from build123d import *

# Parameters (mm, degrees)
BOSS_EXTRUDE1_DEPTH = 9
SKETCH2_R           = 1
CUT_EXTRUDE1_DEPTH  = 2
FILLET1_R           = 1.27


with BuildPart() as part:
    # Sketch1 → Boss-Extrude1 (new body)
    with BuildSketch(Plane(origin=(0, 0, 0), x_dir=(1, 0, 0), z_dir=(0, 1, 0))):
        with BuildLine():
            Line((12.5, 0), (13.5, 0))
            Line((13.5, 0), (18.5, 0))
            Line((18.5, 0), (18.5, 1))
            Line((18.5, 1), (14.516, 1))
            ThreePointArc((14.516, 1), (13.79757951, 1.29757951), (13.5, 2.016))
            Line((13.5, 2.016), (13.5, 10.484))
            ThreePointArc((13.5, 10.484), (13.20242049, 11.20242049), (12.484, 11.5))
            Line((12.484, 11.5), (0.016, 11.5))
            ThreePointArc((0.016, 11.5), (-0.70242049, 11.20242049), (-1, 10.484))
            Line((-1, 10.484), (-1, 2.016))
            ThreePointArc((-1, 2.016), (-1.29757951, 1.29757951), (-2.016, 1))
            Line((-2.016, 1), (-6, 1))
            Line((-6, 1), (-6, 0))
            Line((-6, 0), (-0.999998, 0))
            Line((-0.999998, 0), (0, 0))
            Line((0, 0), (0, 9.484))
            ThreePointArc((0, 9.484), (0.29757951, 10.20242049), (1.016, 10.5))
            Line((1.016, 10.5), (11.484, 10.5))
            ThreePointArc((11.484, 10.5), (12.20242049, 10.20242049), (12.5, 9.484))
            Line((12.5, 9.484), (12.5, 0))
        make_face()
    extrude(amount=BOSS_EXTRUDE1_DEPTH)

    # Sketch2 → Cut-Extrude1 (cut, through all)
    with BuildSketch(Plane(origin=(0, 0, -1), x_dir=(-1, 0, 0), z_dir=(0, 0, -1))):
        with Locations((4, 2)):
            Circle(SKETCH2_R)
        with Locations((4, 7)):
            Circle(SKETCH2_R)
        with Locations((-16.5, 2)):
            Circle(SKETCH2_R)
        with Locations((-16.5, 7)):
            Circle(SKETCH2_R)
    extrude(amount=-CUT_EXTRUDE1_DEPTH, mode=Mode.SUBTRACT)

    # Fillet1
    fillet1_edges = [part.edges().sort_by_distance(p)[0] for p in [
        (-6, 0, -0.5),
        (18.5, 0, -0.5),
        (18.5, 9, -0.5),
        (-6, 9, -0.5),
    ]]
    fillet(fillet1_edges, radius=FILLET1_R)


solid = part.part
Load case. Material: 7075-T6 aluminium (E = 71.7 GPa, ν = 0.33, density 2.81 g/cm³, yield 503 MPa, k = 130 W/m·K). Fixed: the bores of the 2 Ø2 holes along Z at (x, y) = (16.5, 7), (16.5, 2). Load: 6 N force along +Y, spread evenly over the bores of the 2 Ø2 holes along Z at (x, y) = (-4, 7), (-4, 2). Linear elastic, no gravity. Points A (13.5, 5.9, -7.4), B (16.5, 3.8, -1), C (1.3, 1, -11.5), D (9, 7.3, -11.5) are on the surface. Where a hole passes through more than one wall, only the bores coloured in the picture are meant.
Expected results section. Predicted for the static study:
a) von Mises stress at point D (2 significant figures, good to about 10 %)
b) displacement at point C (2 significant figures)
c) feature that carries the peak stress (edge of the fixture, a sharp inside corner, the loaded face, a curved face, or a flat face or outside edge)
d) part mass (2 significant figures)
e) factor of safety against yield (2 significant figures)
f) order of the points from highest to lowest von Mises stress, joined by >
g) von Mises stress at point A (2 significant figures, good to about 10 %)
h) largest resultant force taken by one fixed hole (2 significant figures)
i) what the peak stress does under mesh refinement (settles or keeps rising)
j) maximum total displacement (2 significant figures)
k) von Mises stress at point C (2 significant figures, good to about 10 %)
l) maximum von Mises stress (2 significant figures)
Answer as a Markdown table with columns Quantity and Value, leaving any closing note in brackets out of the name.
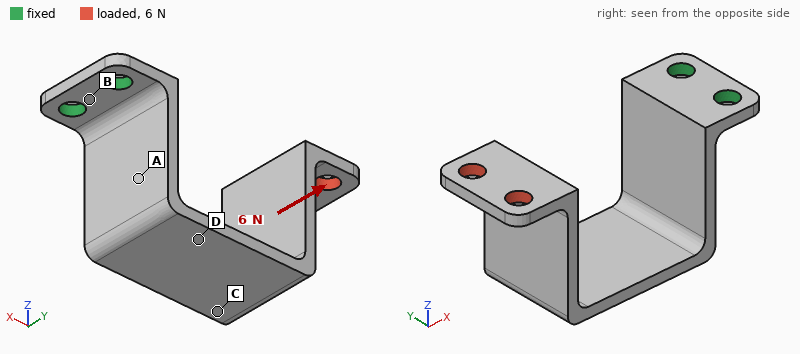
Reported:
| Quantity | Value |
|---|---|
| von Mises stress at point D | 38 MPa |
| displacement at point C | 0.12 mm |
| feature that carries the peak stress | a curved face |
| part mass | 1.1 g |
| factor of safety against yield | 7.9 |
| order of the points from highest to lowest von Mises stress, joined by > | A > D > C > B |
| von Mises stress at point A | 53 MPa |
| largest resultant force taken by one fixed hole | 20 N |
| what the peak stress does under mesh refinement | settles |
| maximum total displacement | 0.32 mm |
| von Mises stress at point C | 27 MPa |
| maximum von Mises stress | 63 MPa |
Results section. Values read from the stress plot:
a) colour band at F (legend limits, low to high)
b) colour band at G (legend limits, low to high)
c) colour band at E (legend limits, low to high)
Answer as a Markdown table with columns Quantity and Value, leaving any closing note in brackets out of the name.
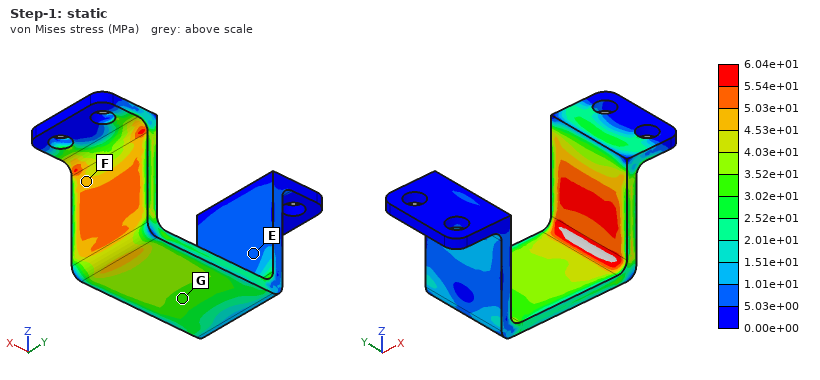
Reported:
| Quantity | Value |
|---|---|
| colour band at F | 4.53e+01 to 5.03e+01 MPa |
| colour band at G | 3.02e+01 to 3.52e+01 MPa |
| colour band at E | 5.03e+00 to 1.01e+01 MPa |
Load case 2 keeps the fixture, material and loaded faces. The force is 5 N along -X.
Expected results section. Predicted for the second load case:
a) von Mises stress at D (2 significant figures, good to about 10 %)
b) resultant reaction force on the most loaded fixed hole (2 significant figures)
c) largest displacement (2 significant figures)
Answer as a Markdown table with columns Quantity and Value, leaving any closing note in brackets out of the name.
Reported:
| Quantity | Value |
|---|---|
| von Mises stress at D | 33 MPa |
| resultant reaction force on the most loaded fixed hole | 2.5 N |
| largest displacement | 0.31 mm |
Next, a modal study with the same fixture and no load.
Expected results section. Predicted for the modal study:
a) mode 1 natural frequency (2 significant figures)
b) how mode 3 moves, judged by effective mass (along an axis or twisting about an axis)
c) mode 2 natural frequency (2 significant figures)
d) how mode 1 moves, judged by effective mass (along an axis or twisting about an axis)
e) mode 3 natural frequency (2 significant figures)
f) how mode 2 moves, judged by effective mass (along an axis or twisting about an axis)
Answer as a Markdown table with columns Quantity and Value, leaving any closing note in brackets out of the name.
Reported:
| Quantity | Value |
|---|---|
| mode 1 natural frequency | 870 Hz |
| how mode 3 moves, judged by effective mass | along X |
| mode 2 natural frequency | 1400 Hz |
| how mode 1 moves, judged by effective mass | along Z |
| mode 3 natural frequency | 2000 Hz |
| how mode 2 moves, judged by effective mass | along Y |
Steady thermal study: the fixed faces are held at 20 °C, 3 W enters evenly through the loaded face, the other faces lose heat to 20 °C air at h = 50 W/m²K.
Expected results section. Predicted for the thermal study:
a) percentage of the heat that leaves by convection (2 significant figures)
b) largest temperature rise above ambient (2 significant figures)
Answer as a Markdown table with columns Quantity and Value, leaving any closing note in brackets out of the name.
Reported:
| Quantity | Value |
|---|---|
| percentage of the heat that leaves by convection | 43 % |
| largest temperature rise above ambient | 69 K |
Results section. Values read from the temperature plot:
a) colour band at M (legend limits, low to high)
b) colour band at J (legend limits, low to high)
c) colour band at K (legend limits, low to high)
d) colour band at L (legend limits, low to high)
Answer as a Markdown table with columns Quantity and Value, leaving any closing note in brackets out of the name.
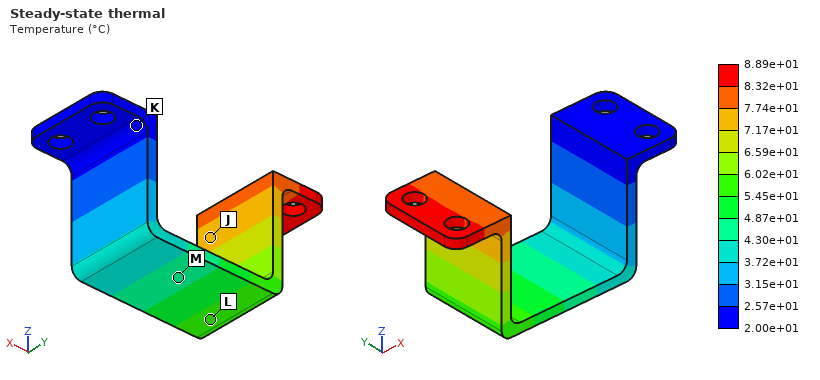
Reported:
| Quantity | Value |
|---|---|
| colour band at M | 4.30e+01 to 4.87e+01 °C |
| colour band at J | 7.17e+01 to 7.74e+01 °C |
| colour band at K | 2.00e+01 to 2.57e+01 °C |
| colour band at L | 5.45e+01 to 6.02e+01 °C |
